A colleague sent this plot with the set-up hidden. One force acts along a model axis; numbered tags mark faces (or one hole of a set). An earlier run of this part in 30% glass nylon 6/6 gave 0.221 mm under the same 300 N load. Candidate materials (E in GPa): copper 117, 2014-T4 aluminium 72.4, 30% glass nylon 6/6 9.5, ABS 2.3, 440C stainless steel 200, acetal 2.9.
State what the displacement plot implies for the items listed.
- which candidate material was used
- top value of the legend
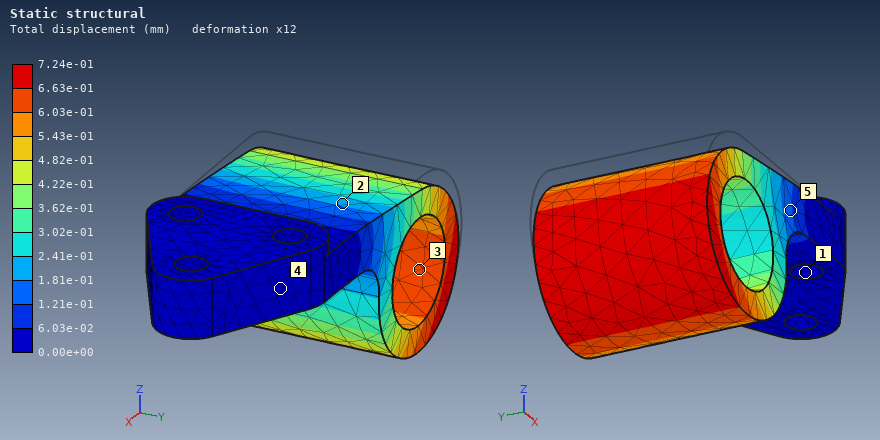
acetal
7.24e-01 mm
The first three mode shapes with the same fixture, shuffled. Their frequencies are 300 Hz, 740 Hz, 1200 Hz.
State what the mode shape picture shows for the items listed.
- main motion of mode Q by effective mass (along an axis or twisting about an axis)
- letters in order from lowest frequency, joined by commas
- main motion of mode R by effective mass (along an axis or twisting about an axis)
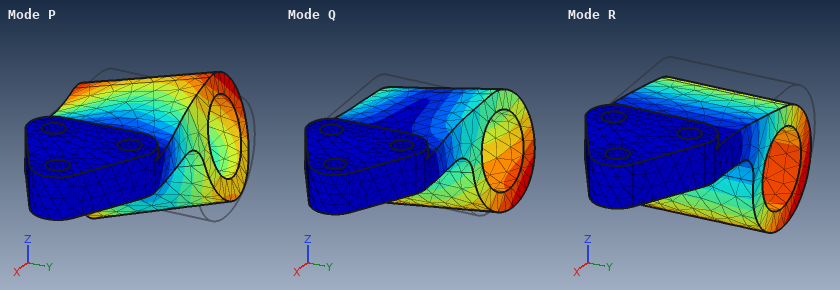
along Y
R, Q, P
along Z
